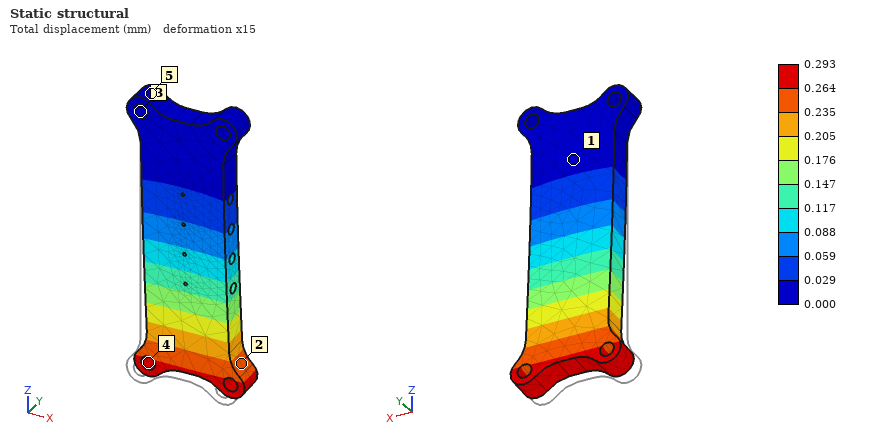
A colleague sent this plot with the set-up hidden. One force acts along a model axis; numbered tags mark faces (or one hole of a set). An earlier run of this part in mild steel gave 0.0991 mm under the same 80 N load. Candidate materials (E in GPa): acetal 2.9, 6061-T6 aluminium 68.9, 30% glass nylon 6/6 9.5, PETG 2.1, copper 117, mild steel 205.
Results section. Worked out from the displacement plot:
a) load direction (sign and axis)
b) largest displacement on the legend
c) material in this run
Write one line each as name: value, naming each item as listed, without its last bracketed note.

load direction: +Y
largest displacement on the legend: 0.293 mm
material in this run: 6061-T6 aluminium
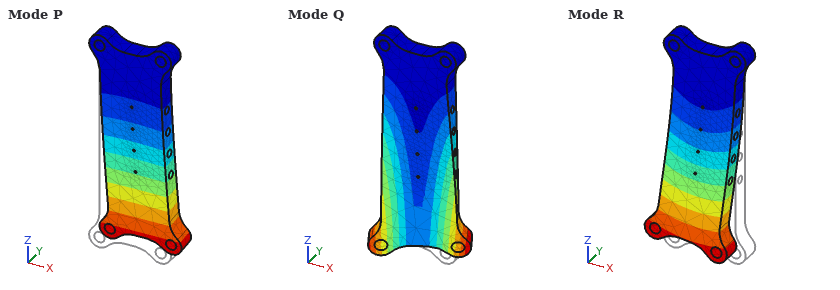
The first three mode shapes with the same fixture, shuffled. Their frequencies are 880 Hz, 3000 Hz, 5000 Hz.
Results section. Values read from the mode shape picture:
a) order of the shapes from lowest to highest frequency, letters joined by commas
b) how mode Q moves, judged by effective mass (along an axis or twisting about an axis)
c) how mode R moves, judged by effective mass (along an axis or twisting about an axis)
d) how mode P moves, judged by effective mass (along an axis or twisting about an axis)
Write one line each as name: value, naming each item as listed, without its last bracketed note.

order of the shapes from lowest to highest frequency, letters joined by commas: P, R, Q
how mode Q moves, judged by effective mass: twisting about Z
how mode R moves, judged by effective mass: along X
how mode P moves, judged by effective mass: along Y
